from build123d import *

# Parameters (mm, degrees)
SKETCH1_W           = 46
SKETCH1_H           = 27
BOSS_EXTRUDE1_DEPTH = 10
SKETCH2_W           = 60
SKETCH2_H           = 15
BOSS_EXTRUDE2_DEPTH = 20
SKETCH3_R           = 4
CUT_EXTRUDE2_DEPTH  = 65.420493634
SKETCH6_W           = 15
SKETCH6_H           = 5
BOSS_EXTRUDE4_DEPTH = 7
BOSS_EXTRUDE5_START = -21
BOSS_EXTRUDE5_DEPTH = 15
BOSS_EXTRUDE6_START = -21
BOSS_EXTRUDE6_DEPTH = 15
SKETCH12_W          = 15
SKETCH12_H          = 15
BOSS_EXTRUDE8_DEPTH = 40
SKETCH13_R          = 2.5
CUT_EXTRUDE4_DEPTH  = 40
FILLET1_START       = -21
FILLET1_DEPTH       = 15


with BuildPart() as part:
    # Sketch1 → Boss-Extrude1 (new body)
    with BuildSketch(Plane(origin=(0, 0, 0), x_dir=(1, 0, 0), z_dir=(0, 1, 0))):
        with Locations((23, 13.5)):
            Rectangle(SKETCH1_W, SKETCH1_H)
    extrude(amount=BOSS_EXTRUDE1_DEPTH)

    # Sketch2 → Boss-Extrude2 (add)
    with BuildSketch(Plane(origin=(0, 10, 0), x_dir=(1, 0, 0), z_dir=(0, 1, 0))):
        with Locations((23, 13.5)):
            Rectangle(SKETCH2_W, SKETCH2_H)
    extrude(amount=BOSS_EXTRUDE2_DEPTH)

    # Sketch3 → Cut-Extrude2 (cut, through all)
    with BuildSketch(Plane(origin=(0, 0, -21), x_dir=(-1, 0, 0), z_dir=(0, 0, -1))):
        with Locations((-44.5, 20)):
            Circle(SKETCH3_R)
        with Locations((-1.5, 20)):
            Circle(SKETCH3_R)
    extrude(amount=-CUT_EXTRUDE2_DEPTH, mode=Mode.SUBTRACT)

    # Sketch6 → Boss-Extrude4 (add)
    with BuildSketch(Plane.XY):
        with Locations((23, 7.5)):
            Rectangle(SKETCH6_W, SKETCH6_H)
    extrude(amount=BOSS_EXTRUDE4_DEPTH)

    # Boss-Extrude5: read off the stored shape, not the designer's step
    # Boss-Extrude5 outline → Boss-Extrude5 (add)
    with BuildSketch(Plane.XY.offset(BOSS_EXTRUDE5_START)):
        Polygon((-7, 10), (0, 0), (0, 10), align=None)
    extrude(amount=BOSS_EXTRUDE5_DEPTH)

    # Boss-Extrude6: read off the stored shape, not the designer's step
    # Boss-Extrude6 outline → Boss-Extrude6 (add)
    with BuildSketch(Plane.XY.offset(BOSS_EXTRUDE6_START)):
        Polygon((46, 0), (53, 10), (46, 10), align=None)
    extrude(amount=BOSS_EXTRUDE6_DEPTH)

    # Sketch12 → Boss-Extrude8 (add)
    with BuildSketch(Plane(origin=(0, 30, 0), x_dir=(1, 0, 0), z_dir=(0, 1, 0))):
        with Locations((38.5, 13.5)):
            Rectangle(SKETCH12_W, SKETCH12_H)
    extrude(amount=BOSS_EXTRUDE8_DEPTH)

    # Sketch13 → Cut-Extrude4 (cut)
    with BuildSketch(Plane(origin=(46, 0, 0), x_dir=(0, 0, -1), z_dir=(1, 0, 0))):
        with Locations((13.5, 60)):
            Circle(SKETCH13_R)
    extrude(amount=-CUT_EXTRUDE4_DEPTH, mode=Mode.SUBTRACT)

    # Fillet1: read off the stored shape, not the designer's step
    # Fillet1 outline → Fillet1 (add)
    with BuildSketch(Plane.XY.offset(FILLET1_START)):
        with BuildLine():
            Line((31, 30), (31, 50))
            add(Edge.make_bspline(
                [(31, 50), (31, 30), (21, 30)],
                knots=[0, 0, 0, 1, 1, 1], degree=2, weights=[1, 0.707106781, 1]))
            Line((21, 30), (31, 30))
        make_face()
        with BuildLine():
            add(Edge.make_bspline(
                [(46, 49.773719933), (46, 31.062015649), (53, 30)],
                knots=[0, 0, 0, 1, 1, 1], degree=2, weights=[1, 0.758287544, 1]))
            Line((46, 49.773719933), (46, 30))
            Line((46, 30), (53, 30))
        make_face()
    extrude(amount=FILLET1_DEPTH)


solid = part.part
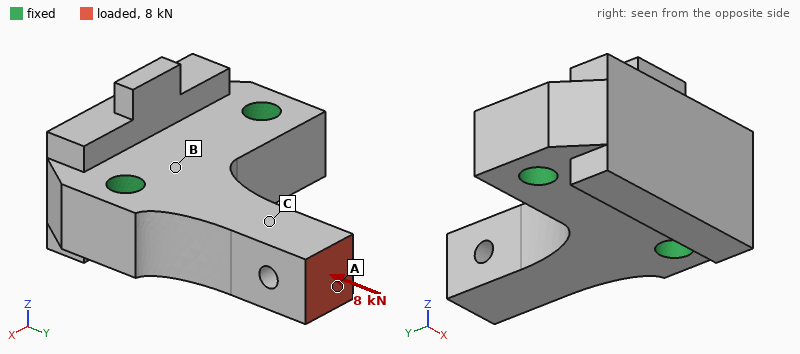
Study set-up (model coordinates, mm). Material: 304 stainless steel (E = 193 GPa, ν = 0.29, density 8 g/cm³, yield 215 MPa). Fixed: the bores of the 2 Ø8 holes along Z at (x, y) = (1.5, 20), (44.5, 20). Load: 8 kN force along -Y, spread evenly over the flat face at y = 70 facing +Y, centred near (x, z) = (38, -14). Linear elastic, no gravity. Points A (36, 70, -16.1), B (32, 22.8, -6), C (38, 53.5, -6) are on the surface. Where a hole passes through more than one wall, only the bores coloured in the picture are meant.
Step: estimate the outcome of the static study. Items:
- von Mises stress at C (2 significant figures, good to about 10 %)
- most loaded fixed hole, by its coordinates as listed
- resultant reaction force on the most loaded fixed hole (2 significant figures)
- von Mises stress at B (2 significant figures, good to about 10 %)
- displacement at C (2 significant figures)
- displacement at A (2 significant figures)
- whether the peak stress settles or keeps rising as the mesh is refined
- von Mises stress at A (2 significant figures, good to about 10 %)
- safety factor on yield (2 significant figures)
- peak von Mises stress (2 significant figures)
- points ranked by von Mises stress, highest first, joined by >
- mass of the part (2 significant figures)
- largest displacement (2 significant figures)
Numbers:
45 MPa
(44.5, 20)
6.9 kN
11 MPa
5.4 µm
9.3 µm
settles
30 MPa
1.8
120 MPa
C > A > B
320 g
9.6 µm
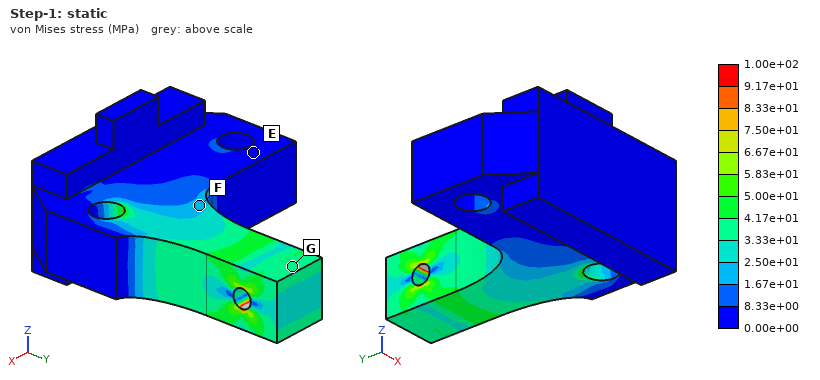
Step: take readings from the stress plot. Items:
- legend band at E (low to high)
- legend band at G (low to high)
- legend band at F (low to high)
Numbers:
0.00e+00 to 8.33e+00 MPa
3.33e+01 to 4.17e+01 MPa
1.67e+01 to 2.50e+01 MPa
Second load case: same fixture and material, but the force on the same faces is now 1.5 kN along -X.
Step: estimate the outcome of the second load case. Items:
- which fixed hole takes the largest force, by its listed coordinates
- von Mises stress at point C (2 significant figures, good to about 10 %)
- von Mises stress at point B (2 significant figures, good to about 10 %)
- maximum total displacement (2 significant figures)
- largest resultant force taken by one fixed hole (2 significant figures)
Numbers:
(44.5, 20)
17 MPa
13 MPa
37 µm
1.9 kN
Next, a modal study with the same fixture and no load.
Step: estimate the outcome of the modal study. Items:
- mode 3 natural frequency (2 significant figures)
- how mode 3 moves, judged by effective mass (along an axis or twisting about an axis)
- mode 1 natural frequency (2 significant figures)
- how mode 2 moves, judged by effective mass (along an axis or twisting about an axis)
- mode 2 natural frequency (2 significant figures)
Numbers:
15 kHz
along Z
5600 Hz
along X
7800 Hz
